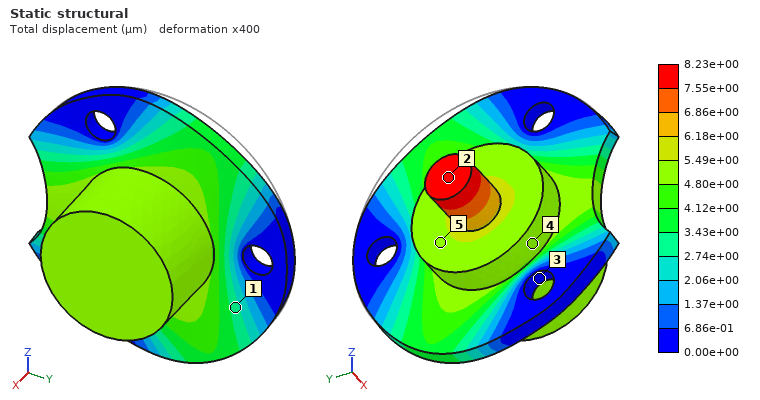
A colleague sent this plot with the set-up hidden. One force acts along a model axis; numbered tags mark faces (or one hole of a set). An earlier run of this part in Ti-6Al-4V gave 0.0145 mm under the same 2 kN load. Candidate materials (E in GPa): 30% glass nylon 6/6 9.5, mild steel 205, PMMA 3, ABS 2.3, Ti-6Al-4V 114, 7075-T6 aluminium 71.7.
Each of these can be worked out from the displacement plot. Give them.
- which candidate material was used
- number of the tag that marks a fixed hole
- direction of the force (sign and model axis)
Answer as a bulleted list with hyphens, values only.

- mild steel
- 3
- +X
